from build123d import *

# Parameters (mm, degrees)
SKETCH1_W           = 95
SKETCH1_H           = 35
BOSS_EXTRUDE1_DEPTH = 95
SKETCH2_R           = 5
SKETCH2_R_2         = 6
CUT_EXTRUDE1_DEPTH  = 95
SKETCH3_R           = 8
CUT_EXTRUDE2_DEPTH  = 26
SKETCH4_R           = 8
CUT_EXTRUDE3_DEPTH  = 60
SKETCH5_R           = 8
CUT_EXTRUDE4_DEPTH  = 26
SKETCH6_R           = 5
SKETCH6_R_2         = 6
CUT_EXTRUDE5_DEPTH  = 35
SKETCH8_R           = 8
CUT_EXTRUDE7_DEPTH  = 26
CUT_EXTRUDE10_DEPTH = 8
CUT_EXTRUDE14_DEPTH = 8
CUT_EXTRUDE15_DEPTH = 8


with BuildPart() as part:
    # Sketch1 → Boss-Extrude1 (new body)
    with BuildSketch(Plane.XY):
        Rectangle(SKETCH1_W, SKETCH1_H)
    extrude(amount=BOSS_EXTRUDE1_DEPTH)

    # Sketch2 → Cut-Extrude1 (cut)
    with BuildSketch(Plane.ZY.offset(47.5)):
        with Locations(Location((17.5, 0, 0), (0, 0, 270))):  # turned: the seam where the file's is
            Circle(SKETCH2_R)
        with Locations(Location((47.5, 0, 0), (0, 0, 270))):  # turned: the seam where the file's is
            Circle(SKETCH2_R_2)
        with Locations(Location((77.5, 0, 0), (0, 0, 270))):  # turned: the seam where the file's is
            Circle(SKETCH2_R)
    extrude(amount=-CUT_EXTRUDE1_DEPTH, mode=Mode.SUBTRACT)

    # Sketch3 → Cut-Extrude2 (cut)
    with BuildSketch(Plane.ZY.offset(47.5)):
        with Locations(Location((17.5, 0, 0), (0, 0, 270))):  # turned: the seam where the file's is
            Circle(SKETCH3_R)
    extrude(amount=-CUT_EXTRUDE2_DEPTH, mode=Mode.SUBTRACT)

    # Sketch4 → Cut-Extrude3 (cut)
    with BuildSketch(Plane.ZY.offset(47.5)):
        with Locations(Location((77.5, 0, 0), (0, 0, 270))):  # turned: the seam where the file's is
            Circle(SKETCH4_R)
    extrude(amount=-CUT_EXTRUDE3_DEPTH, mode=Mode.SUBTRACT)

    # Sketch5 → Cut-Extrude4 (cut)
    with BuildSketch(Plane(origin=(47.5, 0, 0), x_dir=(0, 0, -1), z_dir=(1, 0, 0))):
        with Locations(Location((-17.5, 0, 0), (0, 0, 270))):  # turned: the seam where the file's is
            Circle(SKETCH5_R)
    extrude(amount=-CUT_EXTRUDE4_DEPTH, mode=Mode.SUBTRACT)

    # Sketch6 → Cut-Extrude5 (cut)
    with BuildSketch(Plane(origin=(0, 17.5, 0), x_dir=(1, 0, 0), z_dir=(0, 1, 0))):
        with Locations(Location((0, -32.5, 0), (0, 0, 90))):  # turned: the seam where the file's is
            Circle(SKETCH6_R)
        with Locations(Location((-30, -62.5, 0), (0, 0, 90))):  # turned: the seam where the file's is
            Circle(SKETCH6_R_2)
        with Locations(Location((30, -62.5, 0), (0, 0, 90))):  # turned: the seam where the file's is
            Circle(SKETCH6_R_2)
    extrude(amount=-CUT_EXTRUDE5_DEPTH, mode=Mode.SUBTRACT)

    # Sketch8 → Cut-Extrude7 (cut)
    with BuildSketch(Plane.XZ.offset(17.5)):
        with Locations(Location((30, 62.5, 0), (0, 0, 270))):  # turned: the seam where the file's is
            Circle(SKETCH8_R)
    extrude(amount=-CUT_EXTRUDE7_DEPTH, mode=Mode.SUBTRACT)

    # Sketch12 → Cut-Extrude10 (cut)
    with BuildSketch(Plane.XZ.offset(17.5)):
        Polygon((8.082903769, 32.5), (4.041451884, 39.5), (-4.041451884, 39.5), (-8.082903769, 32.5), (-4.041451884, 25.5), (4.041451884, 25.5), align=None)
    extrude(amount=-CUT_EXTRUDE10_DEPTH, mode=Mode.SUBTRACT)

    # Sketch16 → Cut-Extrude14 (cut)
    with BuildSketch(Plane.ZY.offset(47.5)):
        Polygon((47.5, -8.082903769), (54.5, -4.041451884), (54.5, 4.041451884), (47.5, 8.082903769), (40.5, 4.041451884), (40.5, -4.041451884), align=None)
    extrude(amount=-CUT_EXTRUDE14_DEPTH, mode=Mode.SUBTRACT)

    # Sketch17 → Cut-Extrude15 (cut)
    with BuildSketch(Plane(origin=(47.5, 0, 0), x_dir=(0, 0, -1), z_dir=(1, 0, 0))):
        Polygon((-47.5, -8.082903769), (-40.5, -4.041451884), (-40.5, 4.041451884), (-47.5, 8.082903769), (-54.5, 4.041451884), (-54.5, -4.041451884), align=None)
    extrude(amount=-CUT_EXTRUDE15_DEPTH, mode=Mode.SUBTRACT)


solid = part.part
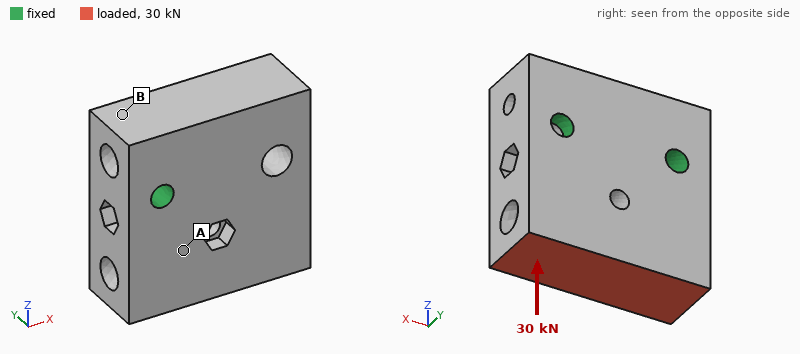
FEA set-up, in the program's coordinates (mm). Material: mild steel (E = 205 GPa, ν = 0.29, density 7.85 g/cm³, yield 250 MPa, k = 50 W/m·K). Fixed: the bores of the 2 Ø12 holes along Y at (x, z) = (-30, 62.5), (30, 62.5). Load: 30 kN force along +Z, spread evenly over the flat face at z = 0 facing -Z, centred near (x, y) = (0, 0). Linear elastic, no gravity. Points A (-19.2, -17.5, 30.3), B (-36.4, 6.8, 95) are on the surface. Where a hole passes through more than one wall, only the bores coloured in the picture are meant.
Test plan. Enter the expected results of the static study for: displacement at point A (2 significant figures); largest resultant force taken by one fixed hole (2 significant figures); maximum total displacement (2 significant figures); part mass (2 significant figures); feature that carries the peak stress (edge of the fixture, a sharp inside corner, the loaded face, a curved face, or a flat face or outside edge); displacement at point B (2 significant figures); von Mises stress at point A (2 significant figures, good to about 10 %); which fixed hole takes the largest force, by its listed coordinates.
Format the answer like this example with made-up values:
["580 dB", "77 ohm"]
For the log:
["5.6 µm", "16 kN", "15 µm", "2.1 kg", "edge of the fixture", "2.3 µm", "19 MPa", "(-30, 62.5)"]
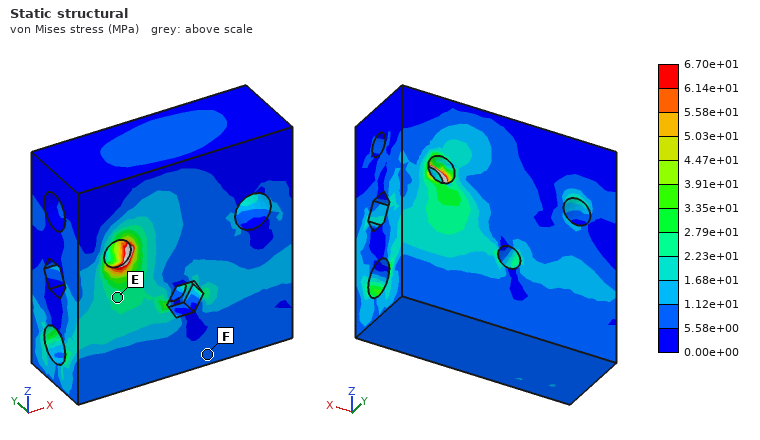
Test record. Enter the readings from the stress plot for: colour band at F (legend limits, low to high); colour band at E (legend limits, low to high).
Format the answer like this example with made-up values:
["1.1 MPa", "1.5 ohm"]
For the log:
["5.58e+00 to 1.12e+01 MPa", "2.23e+01 to 2.79e+01 MPa"]
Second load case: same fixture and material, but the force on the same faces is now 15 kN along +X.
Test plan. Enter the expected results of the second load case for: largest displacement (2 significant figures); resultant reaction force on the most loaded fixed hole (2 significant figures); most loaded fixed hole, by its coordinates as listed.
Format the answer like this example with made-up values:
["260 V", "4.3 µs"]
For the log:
["20 µm", "17 kN", "(-30, 62.5)"]
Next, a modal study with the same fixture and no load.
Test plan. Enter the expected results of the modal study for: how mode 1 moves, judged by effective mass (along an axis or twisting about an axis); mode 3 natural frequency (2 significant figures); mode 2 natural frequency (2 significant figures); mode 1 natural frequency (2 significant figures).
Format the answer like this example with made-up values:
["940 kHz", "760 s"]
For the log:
["along Y", "7900 Hz", "7400 Hz", "3900 Hz"]
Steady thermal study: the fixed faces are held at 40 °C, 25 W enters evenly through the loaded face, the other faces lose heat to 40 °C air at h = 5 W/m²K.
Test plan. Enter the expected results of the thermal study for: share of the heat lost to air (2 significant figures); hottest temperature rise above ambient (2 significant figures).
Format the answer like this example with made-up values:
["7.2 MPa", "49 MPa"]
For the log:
["4.2 %", "14 K"]
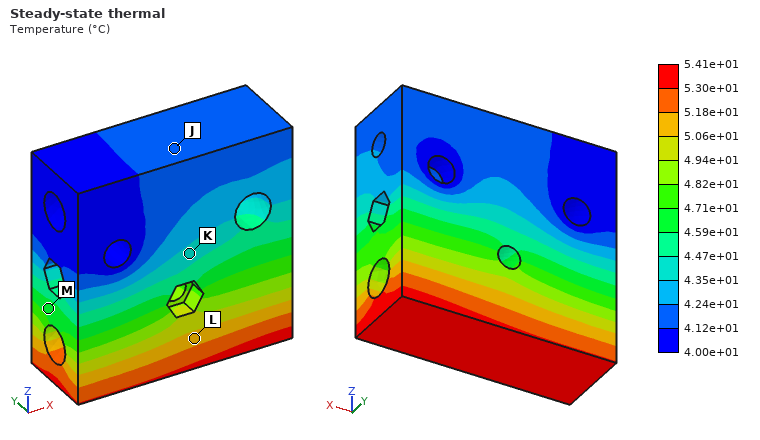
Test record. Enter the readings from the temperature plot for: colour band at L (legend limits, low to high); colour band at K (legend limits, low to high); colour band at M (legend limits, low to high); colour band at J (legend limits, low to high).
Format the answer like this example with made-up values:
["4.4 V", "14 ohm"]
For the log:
["5.06e+01 to 5.18e+01 °C", "4.35e+01 to 4.47e+01 °C", "4.59e+01 to 4.71e+01 °C", "4.12e+01 to 4.24e+01 °C"]
